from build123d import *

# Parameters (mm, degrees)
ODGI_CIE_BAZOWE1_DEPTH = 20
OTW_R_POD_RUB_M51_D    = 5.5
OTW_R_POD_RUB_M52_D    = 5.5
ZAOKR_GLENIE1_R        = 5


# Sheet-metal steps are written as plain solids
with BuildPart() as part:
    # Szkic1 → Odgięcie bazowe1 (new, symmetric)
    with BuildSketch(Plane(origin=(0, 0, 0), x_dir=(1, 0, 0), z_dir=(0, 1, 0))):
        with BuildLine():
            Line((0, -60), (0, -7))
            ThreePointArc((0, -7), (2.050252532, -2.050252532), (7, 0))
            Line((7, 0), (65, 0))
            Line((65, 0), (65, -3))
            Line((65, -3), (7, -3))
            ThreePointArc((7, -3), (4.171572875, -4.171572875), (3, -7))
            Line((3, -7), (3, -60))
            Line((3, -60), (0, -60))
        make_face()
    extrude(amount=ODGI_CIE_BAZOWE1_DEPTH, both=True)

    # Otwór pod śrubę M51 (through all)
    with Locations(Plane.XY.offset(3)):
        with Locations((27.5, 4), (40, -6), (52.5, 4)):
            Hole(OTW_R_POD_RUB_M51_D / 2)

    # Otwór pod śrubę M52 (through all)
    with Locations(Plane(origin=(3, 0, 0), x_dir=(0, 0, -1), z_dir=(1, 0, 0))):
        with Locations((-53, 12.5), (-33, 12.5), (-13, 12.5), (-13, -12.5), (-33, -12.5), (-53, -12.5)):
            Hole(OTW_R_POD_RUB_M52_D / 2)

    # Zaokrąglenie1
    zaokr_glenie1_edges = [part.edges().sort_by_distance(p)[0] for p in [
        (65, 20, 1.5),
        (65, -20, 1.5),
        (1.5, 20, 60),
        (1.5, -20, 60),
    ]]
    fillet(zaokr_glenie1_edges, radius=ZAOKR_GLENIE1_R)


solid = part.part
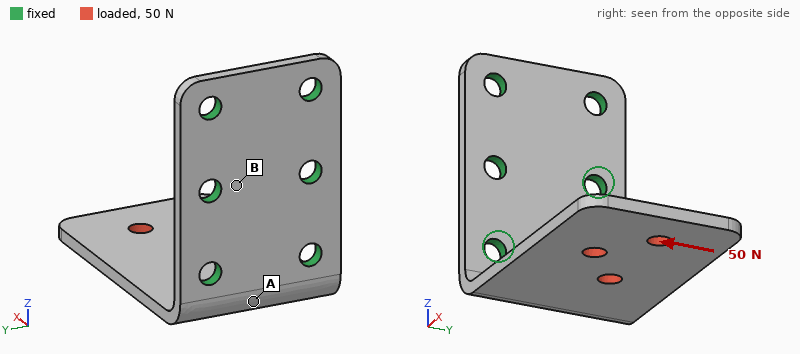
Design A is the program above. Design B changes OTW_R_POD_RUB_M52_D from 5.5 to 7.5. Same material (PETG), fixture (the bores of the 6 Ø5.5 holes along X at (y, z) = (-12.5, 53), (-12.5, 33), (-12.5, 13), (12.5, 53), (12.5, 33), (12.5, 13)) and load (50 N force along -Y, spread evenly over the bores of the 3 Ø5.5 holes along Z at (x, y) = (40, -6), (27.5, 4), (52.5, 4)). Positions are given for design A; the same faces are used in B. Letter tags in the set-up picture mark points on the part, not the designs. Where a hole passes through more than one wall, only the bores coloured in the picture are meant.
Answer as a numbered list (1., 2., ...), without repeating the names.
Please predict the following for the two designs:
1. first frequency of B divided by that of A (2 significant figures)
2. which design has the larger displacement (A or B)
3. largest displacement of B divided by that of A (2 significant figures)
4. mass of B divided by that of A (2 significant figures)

1. 1.0
2. A
3. 0.78
4. 0.97
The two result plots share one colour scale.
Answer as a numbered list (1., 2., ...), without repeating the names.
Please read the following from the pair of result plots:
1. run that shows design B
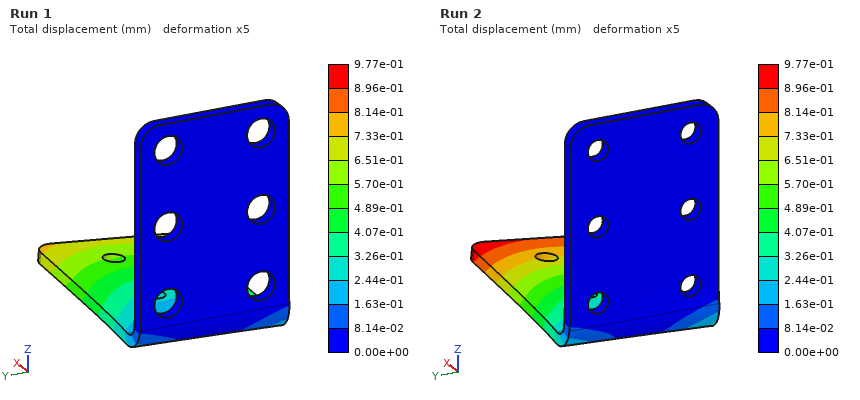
1. Run 1
